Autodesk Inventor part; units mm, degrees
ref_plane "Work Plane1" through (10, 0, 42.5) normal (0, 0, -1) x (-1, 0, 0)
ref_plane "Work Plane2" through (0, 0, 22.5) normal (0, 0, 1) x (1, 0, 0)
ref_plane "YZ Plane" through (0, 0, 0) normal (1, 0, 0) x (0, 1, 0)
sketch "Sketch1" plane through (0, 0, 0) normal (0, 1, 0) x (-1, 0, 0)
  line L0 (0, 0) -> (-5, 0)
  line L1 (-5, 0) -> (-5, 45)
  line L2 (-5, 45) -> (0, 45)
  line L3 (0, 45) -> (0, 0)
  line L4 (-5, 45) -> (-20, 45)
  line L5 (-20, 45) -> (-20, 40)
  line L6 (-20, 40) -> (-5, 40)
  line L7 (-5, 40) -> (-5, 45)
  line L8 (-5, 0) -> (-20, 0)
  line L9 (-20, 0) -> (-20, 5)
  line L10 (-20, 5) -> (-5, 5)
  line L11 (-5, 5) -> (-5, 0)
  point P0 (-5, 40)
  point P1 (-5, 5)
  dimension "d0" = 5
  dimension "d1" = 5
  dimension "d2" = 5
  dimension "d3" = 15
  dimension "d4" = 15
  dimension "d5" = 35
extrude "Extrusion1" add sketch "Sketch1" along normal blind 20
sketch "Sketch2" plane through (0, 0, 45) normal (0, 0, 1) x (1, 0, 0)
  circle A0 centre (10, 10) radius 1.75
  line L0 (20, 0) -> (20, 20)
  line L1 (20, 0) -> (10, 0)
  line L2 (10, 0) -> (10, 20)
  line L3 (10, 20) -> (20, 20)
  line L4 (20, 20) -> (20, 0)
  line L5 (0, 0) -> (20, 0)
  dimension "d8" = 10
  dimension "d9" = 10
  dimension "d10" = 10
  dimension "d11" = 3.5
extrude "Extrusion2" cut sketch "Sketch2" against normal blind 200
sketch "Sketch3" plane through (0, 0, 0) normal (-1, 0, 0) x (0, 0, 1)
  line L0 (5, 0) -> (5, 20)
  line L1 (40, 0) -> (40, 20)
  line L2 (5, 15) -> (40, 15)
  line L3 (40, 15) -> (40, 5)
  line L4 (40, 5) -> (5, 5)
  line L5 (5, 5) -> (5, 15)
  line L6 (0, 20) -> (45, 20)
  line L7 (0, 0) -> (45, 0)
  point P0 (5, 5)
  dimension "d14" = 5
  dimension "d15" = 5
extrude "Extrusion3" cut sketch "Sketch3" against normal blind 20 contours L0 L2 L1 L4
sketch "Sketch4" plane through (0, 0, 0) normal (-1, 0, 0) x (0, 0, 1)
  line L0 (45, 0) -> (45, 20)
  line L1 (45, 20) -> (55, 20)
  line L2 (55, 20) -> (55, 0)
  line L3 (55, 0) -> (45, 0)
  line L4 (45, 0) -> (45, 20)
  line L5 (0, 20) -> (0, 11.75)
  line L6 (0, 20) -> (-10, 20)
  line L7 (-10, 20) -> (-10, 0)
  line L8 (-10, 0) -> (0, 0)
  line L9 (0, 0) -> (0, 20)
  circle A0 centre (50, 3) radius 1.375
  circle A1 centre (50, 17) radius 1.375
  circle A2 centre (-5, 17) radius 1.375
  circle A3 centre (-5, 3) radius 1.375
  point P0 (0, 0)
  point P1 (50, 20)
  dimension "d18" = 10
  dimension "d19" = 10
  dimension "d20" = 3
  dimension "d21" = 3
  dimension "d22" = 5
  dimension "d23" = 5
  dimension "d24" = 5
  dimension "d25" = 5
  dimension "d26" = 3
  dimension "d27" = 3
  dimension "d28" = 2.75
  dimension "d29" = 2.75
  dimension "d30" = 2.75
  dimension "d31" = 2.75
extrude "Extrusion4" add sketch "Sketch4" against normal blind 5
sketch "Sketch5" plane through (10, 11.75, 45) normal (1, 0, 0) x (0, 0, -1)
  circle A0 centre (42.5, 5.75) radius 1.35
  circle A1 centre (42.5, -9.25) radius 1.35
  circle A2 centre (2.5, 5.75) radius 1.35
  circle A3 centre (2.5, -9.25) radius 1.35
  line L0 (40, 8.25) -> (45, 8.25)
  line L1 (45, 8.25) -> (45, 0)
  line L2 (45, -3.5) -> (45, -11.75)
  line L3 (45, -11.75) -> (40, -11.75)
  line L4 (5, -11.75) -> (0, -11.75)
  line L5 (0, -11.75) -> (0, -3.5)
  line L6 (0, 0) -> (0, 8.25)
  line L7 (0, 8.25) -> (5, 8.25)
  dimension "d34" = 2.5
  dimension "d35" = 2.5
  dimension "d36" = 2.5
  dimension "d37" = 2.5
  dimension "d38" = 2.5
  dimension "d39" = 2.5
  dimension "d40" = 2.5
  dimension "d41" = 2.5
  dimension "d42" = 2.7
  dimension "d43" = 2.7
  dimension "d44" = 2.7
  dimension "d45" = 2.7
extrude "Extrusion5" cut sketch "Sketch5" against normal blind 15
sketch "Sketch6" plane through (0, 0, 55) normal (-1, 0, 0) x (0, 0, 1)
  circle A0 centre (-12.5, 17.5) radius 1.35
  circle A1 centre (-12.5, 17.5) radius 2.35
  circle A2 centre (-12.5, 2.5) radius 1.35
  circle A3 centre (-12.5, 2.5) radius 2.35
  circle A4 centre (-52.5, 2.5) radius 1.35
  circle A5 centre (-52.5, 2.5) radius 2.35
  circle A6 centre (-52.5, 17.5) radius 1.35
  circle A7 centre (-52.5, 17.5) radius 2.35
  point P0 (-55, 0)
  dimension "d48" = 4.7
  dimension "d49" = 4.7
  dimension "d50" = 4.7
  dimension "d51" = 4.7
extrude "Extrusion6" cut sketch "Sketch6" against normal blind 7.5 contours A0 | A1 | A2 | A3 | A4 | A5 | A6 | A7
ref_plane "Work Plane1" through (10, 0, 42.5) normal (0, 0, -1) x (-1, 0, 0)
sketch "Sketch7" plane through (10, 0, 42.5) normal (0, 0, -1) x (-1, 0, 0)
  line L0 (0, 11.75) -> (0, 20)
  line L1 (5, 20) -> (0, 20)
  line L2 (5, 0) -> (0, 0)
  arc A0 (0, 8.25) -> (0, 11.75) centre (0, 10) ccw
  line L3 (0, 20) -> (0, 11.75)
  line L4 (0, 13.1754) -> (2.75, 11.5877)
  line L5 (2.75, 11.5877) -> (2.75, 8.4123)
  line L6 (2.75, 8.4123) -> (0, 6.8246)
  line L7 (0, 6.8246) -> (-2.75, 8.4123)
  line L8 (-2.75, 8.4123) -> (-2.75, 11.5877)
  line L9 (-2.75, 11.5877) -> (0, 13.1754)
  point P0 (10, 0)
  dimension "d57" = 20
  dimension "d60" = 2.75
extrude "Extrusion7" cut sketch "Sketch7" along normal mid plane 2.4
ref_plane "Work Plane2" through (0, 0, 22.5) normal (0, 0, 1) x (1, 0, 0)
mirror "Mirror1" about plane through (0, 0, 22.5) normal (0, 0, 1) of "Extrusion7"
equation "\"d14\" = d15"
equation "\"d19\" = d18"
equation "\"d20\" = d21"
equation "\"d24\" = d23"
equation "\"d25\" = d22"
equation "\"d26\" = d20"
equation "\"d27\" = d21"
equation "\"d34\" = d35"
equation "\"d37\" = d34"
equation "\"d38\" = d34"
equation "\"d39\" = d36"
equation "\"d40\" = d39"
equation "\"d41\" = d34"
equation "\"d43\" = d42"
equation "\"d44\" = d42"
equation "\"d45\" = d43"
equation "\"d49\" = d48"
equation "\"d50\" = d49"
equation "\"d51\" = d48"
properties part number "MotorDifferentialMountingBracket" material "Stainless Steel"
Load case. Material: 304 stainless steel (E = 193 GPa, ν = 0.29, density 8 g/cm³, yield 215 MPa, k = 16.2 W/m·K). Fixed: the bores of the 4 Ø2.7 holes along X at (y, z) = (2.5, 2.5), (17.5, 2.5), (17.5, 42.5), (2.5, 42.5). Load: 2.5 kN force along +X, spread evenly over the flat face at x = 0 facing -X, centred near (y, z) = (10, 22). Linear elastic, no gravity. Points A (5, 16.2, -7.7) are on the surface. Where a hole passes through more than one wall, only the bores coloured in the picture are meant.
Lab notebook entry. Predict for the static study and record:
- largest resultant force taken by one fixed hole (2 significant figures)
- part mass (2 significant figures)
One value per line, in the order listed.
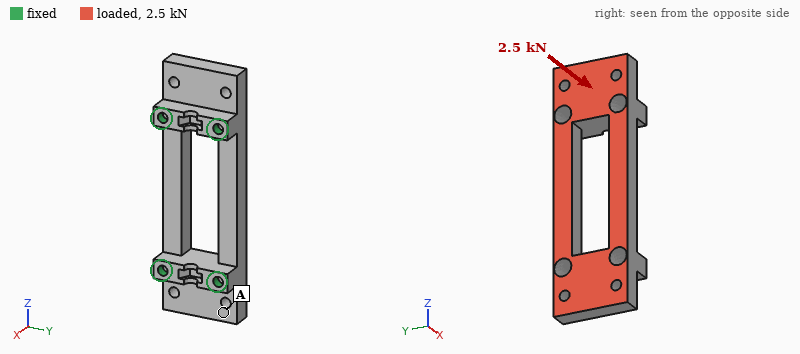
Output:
660 N
40 g
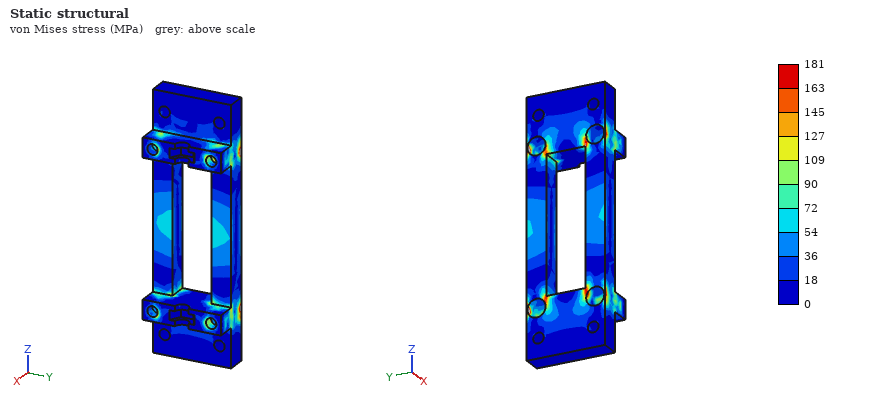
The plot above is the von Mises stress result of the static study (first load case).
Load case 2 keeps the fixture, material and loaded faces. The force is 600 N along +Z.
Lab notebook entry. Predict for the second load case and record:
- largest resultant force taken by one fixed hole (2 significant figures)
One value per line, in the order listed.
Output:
150 N
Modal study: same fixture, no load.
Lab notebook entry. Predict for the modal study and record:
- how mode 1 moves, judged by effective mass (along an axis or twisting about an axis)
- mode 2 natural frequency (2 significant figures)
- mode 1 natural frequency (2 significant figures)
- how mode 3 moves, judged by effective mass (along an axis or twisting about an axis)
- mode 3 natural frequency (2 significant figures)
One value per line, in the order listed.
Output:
along Z
10 kHz
9300 Hz
twisting about Z
12 kHz
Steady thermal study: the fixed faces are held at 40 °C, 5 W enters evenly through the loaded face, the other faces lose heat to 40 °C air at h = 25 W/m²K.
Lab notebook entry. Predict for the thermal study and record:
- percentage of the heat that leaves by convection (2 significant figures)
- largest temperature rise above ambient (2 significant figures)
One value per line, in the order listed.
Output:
27 %
26 K
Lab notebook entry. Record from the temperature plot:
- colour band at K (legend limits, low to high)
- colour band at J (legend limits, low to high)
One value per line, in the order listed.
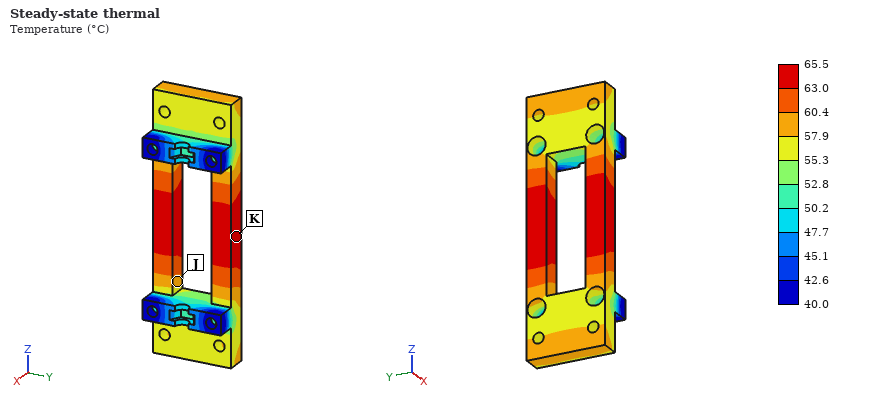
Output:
63.0 to 65.5 °C
57.9 to 60.4 °C
